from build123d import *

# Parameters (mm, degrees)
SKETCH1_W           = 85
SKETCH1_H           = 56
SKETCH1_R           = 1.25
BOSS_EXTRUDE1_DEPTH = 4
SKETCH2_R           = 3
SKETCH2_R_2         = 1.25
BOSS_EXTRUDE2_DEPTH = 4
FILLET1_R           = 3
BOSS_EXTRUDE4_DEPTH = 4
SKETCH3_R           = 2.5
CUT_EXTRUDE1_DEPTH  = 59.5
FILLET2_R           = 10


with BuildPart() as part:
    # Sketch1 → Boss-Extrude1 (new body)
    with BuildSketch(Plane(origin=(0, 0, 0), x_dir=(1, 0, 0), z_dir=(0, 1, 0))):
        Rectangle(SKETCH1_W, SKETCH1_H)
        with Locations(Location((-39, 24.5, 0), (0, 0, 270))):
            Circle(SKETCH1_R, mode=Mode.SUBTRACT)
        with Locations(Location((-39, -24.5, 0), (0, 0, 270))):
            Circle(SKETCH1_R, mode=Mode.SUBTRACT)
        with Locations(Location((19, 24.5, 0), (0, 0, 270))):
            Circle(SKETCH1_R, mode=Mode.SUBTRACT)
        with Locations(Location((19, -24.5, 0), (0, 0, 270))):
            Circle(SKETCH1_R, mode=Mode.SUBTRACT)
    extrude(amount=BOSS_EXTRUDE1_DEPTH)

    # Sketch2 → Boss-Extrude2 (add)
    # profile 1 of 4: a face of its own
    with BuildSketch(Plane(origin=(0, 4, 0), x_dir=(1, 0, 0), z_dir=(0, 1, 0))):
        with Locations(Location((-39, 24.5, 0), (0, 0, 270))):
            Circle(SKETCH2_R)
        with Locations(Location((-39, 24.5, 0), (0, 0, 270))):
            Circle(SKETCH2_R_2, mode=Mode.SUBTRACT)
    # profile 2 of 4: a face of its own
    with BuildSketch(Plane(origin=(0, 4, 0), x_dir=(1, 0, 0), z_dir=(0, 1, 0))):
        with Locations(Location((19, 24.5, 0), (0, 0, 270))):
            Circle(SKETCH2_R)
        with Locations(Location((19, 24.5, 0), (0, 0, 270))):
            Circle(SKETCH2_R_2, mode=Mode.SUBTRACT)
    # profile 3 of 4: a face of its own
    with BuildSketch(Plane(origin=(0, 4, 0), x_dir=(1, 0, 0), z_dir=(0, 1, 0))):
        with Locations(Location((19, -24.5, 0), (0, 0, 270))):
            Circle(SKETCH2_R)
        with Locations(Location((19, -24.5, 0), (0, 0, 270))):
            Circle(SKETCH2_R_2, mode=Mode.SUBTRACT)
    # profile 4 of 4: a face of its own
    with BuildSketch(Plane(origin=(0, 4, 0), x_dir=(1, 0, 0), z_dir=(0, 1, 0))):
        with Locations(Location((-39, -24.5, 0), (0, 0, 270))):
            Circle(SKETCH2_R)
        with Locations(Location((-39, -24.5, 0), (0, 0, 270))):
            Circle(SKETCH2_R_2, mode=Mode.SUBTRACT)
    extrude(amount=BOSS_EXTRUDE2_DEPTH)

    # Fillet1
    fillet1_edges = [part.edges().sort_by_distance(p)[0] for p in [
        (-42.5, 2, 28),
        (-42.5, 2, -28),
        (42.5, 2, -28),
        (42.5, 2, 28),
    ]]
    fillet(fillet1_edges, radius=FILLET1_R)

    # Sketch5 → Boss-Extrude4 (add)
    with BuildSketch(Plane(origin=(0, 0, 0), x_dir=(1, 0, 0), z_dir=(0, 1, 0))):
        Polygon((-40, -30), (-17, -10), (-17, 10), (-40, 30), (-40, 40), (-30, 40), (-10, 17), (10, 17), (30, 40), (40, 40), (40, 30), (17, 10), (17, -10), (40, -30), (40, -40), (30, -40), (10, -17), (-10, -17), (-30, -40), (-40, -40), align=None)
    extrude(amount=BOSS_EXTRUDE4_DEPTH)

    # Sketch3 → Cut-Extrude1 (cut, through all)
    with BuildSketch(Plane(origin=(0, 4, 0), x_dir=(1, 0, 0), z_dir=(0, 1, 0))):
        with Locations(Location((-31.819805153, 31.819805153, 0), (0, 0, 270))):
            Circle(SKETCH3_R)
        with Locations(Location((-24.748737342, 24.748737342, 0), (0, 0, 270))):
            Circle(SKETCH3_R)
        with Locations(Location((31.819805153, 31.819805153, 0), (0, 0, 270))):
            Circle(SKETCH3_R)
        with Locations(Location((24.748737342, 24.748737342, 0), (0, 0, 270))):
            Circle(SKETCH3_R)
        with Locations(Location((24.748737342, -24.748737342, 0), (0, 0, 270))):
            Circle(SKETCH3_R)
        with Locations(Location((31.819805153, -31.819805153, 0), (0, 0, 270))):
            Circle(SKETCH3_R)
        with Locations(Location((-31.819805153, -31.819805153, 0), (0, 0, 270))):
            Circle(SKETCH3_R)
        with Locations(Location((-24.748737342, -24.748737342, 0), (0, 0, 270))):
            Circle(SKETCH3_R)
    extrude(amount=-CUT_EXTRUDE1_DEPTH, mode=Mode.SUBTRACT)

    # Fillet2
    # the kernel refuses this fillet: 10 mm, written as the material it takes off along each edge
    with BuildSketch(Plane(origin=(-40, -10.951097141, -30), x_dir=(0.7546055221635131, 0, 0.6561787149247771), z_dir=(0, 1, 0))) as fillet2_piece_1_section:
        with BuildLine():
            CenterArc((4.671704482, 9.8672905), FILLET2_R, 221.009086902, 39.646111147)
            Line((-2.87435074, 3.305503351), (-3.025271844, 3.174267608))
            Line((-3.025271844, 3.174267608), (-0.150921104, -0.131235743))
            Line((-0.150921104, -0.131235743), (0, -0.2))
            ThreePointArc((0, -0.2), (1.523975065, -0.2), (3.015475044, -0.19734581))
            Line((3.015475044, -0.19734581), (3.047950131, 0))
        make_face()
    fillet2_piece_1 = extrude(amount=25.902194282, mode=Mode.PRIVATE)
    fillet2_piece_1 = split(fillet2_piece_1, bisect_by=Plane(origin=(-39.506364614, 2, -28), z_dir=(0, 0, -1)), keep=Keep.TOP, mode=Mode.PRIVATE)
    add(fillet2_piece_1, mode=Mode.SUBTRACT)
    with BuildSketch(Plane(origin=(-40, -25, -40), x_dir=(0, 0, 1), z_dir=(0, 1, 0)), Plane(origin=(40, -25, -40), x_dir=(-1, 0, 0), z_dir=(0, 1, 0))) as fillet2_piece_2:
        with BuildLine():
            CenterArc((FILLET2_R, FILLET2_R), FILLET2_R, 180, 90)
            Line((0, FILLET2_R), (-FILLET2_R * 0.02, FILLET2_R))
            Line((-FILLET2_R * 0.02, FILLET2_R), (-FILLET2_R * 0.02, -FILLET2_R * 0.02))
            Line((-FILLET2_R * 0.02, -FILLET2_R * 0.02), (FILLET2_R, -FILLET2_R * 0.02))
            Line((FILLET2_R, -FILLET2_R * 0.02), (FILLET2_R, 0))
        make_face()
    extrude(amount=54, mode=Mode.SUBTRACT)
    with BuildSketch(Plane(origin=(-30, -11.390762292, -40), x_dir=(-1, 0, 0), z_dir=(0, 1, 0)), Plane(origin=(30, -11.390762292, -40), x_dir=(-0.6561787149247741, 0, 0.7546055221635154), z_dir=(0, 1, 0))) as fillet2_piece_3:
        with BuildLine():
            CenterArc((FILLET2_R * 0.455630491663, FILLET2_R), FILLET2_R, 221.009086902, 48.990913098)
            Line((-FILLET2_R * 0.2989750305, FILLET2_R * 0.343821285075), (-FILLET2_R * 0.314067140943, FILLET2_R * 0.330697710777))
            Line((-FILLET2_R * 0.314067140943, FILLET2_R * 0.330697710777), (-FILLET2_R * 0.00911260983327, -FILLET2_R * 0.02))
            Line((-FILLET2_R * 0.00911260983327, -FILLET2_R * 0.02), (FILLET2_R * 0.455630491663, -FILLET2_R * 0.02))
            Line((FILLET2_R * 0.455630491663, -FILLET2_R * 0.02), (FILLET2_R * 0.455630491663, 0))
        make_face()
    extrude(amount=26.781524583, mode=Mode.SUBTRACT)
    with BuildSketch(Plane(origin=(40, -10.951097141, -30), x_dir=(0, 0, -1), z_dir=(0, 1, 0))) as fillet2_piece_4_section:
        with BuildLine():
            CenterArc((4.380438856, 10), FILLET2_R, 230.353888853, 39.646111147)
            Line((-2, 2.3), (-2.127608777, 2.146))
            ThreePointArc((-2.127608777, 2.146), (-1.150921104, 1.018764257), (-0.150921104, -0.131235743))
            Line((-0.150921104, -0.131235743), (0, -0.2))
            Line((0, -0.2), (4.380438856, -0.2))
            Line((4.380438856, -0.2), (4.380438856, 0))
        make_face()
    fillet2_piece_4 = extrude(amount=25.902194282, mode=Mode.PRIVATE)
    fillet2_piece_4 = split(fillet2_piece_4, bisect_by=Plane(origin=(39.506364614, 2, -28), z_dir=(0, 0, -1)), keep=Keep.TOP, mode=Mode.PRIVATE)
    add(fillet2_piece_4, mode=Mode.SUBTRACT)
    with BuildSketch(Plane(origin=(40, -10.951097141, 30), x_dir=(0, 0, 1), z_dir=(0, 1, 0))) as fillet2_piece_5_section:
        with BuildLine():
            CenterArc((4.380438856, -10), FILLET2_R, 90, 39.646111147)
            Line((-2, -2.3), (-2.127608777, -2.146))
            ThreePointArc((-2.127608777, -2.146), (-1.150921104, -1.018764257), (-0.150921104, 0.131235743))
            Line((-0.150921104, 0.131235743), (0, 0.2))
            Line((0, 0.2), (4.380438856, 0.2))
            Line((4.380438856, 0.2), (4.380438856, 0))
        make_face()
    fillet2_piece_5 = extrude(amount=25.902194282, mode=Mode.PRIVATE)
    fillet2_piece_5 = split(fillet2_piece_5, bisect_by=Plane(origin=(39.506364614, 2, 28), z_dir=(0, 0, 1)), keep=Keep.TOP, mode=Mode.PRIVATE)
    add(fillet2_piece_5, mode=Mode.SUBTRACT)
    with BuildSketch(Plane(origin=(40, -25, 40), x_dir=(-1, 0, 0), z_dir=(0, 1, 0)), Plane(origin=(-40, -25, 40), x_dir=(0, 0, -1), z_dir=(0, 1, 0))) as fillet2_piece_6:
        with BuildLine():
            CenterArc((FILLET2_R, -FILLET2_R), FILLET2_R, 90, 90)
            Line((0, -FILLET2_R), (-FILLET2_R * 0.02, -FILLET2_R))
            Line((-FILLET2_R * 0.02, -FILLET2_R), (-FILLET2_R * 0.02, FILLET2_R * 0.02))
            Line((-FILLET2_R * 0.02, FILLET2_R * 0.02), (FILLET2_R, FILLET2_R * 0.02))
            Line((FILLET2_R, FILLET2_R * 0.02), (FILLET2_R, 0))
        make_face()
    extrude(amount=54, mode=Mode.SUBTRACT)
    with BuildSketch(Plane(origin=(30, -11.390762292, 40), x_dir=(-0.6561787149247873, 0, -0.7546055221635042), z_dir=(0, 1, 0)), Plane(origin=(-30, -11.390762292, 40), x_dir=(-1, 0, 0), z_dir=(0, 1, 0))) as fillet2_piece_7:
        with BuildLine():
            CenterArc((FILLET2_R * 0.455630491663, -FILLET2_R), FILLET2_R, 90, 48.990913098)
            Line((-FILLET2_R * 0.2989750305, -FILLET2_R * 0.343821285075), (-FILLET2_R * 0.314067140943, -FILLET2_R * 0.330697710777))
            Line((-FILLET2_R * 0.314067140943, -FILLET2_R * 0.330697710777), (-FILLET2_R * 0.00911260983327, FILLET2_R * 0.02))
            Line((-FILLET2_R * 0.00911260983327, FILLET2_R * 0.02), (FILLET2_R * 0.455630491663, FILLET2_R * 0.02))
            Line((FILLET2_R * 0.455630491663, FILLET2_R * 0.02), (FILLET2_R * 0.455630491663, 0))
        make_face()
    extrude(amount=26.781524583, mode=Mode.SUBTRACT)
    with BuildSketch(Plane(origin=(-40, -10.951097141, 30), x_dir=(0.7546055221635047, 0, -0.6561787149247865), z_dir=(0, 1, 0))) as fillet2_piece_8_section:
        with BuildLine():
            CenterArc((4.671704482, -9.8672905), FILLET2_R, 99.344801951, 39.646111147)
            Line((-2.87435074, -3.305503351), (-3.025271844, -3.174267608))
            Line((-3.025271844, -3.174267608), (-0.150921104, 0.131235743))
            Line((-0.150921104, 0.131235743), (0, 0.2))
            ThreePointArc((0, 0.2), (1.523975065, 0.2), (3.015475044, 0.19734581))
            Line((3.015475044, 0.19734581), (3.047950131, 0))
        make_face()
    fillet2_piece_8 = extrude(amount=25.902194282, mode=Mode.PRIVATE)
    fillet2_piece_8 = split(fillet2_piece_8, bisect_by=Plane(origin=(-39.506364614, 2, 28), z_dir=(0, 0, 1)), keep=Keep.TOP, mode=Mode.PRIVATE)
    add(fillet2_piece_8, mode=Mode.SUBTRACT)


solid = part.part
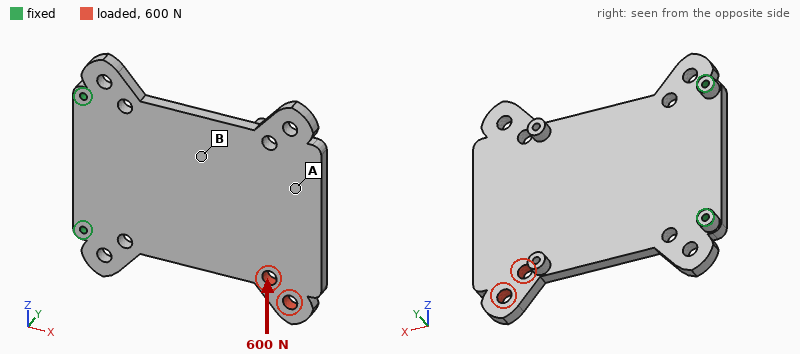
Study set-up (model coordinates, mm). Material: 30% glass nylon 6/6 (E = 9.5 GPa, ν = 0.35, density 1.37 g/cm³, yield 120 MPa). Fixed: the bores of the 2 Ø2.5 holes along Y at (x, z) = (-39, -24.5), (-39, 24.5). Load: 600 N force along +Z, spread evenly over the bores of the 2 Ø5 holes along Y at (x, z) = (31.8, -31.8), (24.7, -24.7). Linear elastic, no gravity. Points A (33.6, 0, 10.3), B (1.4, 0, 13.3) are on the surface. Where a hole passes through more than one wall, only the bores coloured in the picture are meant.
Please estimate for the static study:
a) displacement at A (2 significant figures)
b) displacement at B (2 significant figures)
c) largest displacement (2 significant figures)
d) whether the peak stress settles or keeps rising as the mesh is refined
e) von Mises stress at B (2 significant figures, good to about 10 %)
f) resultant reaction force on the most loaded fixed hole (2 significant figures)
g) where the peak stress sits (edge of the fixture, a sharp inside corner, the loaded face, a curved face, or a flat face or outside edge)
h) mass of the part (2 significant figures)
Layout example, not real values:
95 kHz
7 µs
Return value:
0.21 mm
0.10 mm
0.26 mm
keeps rising
6.5 MPa
870 N
edge of the fixture
29 g
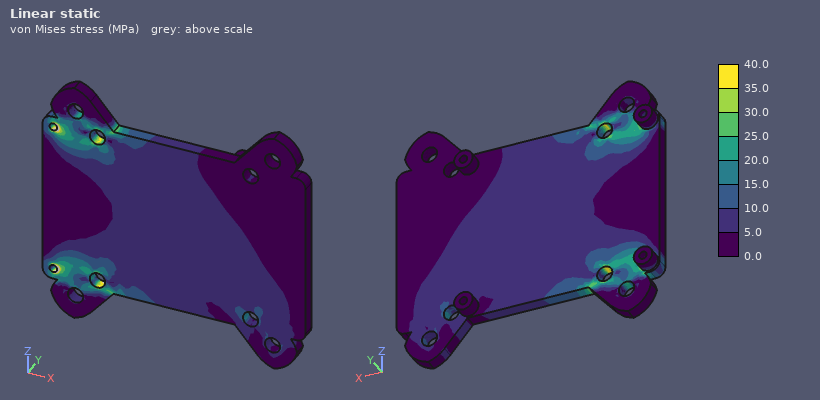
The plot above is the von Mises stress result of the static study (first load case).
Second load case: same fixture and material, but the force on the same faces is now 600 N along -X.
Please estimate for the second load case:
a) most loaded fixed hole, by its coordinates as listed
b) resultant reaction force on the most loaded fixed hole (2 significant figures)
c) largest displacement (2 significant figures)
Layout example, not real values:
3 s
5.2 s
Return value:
(-39, -24.5)
650 N
0.19 mm
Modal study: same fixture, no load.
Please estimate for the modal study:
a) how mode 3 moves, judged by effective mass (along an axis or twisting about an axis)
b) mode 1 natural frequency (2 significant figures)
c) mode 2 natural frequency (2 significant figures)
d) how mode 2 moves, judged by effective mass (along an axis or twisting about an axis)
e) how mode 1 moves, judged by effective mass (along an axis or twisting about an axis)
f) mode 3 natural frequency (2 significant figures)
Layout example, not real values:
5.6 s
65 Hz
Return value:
along Y
210 Hz
680 Hz
twisting about X
along Y
1400 Hz
